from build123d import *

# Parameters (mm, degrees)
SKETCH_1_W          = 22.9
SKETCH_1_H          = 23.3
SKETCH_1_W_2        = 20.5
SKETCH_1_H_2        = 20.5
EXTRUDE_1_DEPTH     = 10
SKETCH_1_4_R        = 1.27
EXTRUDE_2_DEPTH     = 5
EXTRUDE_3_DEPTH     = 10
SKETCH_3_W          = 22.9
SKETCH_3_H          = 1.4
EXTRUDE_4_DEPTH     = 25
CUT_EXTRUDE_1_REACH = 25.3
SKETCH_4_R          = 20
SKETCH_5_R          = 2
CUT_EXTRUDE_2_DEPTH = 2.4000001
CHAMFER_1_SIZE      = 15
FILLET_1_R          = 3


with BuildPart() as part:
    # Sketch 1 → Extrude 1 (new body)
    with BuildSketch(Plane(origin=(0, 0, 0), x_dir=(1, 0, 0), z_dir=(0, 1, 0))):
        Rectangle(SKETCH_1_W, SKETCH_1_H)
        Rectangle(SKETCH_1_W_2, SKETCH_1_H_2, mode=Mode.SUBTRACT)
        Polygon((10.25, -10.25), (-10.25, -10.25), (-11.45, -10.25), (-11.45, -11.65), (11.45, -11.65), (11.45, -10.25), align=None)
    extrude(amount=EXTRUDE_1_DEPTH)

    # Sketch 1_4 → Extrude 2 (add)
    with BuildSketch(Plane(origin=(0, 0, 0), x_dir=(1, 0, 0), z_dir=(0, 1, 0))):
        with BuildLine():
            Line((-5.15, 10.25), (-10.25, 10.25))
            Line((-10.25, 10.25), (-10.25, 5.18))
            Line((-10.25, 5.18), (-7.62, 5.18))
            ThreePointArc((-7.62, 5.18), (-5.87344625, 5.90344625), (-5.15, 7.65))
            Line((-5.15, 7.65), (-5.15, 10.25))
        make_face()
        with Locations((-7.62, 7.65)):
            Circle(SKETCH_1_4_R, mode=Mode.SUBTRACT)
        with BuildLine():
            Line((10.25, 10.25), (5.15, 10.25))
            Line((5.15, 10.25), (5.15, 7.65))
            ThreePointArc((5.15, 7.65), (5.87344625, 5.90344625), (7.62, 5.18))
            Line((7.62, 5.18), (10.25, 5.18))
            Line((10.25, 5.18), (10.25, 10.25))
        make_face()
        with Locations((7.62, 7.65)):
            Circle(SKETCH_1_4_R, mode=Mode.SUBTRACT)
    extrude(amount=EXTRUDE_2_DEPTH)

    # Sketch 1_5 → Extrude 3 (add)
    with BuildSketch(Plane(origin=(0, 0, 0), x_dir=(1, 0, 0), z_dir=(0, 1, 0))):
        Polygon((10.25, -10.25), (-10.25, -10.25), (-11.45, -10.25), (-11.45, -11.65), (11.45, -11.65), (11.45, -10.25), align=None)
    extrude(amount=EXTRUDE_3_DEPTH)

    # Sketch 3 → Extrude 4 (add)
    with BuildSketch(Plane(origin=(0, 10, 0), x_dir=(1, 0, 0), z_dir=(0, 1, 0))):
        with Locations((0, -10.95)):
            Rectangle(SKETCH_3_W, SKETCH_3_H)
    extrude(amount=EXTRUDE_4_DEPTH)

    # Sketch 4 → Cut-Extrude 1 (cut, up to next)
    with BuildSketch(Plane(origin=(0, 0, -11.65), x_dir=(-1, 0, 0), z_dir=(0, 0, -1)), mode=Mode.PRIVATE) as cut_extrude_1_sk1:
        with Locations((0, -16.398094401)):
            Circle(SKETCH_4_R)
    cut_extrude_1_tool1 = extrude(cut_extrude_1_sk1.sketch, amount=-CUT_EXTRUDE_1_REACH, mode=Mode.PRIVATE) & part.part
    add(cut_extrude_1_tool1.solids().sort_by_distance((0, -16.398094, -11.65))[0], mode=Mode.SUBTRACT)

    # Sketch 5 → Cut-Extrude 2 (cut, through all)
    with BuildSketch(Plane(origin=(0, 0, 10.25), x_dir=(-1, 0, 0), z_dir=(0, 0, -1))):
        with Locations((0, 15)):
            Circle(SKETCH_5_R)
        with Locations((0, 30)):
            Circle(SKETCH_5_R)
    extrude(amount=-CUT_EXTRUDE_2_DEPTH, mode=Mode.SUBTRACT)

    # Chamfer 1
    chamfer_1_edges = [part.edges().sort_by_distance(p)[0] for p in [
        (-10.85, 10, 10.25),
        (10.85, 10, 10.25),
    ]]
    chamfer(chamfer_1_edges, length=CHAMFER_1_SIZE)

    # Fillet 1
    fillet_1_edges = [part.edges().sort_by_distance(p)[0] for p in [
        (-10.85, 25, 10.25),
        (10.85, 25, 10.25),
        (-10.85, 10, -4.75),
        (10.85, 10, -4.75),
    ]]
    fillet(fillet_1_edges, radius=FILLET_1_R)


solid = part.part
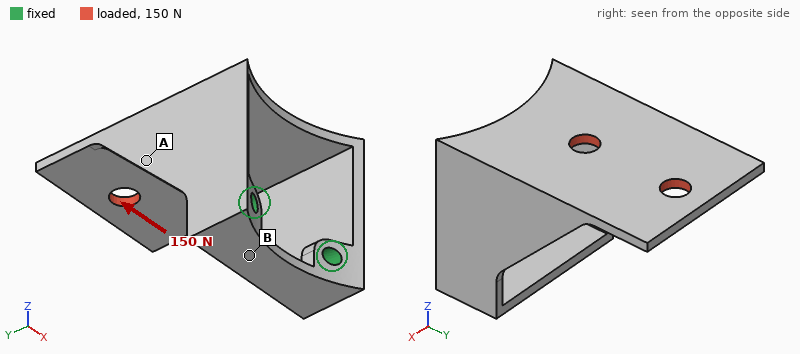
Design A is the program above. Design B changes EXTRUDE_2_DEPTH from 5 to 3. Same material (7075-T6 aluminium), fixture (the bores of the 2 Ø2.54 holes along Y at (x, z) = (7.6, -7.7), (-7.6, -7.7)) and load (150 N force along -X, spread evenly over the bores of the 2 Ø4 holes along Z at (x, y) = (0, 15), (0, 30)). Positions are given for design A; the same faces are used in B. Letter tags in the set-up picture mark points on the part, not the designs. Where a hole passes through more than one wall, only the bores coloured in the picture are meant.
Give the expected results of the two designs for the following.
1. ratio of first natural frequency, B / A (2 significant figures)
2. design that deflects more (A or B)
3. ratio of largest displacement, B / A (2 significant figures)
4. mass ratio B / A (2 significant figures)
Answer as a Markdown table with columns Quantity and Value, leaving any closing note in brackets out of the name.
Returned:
| Quantity | Value |
|---|---|
| ratio of first natural frequency, B / A | 0.85 |
| design that deflects more | B |
| ratio of largest displacement, B / A | 1.6 |
| mass ratio B / A | 0.96 |
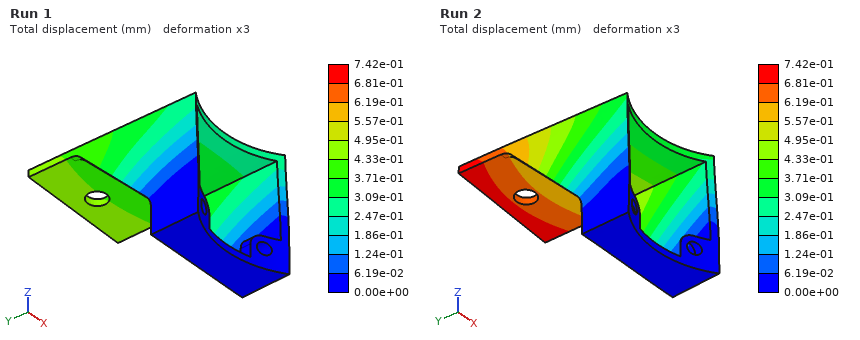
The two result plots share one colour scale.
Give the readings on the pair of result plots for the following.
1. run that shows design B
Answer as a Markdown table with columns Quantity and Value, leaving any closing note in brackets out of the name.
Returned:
| Quantity | Value |
|---|---|
| run that shows design B | Run 2 |
